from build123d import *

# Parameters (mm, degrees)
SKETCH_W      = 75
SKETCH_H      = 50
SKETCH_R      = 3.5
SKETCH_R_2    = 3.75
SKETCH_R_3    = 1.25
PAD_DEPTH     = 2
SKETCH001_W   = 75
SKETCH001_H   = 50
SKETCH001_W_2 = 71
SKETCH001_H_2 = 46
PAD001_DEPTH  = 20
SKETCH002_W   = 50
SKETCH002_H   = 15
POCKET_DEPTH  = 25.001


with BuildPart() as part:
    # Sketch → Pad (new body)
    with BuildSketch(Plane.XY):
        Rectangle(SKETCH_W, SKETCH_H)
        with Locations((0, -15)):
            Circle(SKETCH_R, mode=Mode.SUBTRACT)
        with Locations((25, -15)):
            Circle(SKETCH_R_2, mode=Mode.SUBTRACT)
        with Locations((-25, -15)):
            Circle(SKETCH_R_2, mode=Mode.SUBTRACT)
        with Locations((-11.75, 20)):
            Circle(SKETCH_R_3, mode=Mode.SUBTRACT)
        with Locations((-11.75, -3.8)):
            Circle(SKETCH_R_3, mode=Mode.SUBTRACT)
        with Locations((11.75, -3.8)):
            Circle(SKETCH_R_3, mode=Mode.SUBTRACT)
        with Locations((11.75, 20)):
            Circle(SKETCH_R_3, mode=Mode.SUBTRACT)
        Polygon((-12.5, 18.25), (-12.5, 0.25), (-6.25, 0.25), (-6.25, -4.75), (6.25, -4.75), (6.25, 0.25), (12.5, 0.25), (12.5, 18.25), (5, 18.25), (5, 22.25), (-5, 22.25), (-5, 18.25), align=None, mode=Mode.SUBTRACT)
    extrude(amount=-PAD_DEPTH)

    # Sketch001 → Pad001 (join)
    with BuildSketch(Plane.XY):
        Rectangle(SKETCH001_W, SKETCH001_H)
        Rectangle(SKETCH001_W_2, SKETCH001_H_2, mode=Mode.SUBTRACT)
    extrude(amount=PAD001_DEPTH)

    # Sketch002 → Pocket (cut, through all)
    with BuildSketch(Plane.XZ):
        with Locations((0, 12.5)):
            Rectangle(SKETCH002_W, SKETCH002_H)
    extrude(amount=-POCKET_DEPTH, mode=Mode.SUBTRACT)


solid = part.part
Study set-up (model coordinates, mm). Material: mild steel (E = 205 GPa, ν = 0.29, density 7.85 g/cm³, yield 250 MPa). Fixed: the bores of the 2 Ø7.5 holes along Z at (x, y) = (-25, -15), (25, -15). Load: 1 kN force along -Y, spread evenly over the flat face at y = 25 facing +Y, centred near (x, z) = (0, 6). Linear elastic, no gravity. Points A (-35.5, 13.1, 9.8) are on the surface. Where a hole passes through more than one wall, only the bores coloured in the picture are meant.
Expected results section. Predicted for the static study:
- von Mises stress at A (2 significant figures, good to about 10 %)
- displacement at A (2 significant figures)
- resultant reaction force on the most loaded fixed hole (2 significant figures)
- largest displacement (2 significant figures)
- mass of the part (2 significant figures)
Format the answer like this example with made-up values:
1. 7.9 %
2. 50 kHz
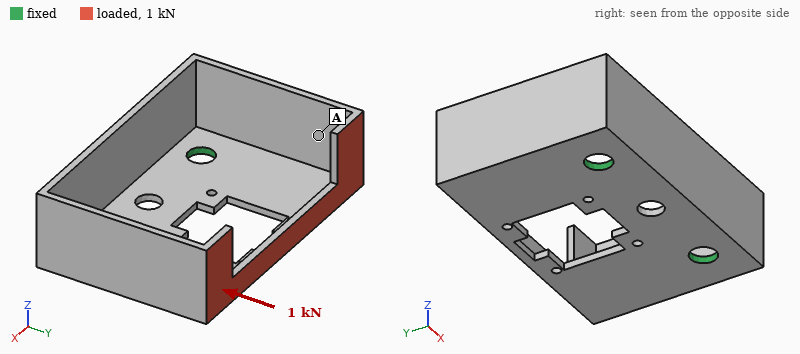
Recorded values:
1. 15 MPa
2. 0.059 mm
3. 500 N
4. 0.10 mm
5. 110 g
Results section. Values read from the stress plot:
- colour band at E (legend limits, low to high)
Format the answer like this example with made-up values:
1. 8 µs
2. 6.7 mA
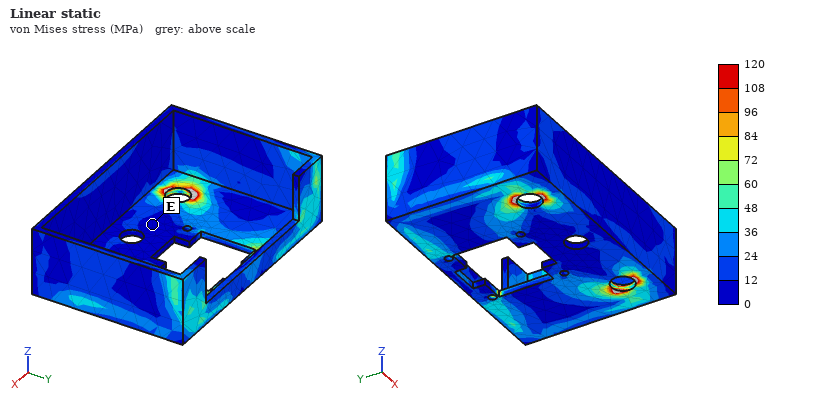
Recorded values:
1. 0 to 12 MPa
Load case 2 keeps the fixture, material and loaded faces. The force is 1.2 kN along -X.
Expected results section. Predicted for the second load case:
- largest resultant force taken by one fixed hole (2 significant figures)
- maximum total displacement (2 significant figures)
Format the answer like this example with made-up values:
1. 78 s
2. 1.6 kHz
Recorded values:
1. 910 N
2. 0.16 mm
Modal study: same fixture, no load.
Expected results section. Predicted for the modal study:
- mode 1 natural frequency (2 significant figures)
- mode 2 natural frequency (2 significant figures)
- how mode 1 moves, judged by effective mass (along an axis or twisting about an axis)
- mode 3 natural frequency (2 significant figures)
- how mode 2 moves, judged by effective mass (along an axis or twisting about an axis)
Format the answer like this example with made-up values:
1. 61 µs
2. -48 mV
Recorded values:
1. 1300 Hz
2. 1400 Hz
3. along Z
4. 3000 Hz
5. twisting about Y
